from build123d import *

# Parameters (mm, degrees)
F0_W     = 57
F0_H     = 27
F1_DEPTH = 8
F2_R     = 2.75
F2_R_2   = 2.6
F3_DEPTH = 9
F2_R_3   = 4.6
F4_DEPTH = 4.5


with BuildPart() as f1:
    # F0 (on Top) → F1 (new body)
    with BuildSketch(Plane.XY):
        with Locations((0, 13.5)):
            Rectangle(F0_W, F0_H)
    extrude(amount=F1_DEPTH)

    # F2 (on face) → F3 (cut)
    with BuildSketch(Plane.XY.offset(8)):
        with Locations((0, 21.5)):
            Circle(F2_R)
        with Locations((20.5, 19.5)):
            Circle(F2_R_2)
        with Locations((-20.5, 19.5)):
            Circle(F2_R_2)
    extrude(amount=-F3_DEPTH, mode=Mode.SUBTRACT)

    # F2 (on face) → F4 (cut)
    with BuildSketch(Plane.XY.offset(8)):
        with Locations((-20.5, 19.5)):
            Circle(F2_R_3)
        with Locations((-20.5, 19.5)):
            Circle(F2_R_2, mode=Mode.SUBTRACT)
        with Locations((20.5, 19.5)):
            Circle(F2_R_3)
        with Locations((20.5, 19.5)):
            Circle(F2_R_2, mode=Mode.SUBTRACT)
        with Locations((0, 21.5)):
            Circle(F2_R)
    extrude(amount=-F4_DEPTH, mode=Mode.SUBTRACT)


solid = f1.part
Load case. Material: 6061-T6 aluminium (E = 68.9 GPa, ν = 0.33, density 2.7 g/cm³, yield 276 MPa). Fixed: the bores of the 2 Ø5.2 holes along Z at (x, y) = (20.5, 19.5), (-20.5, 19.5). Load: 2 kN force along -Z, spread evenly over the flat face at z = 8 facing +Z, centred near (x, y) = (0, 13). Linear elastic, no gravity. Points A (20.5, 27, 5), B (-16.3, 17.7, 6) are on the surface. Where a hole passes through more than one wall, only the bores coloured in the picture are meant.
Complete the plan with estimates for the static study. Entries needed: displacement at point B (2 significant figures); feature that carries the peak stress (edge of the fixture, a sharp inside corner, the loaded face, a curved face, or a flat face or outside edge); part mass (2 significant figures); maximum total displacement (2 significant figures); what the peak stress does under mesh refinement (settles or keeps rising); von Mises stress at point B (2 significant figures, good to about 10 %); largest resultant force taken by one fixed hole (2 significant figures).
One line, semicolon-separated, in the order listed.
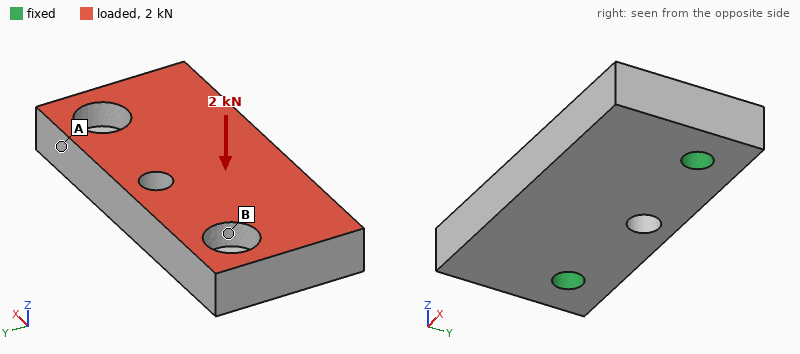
10 µm; edge of the fixture; 31 g; 53 µm; keeps rising; 31 MPa; 1.1 kN
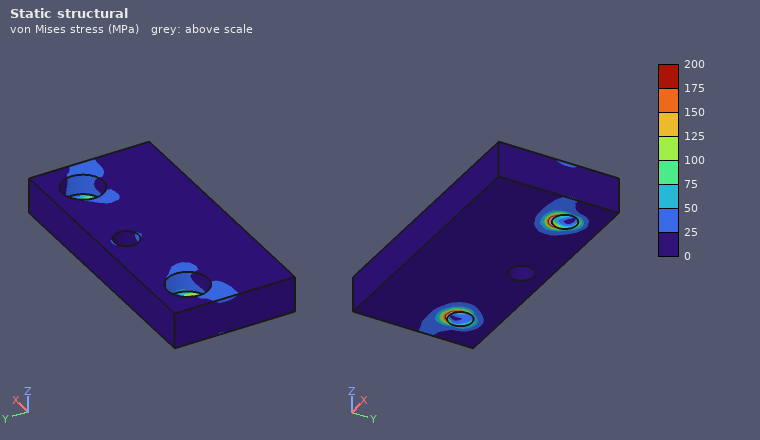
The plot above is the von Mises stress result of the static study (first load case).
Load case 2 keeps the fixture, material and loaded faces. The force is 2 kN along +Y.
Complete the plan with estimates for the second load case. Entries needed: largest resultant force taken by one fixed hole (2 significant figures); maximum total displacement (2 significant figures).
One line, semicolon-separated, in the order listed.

1.0 kN; 43 µm
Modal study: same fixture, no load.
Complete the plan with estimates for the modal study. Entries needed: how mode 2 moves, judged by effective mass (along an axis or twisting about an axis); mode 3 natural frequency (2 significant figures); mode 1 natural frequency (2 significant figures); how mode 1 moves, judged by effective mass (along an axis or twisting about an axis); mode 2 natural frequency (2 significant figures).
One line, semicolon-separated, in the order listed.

twisting about Y; 15 kHz; 6800 Hz; along Z; 13 kHz
